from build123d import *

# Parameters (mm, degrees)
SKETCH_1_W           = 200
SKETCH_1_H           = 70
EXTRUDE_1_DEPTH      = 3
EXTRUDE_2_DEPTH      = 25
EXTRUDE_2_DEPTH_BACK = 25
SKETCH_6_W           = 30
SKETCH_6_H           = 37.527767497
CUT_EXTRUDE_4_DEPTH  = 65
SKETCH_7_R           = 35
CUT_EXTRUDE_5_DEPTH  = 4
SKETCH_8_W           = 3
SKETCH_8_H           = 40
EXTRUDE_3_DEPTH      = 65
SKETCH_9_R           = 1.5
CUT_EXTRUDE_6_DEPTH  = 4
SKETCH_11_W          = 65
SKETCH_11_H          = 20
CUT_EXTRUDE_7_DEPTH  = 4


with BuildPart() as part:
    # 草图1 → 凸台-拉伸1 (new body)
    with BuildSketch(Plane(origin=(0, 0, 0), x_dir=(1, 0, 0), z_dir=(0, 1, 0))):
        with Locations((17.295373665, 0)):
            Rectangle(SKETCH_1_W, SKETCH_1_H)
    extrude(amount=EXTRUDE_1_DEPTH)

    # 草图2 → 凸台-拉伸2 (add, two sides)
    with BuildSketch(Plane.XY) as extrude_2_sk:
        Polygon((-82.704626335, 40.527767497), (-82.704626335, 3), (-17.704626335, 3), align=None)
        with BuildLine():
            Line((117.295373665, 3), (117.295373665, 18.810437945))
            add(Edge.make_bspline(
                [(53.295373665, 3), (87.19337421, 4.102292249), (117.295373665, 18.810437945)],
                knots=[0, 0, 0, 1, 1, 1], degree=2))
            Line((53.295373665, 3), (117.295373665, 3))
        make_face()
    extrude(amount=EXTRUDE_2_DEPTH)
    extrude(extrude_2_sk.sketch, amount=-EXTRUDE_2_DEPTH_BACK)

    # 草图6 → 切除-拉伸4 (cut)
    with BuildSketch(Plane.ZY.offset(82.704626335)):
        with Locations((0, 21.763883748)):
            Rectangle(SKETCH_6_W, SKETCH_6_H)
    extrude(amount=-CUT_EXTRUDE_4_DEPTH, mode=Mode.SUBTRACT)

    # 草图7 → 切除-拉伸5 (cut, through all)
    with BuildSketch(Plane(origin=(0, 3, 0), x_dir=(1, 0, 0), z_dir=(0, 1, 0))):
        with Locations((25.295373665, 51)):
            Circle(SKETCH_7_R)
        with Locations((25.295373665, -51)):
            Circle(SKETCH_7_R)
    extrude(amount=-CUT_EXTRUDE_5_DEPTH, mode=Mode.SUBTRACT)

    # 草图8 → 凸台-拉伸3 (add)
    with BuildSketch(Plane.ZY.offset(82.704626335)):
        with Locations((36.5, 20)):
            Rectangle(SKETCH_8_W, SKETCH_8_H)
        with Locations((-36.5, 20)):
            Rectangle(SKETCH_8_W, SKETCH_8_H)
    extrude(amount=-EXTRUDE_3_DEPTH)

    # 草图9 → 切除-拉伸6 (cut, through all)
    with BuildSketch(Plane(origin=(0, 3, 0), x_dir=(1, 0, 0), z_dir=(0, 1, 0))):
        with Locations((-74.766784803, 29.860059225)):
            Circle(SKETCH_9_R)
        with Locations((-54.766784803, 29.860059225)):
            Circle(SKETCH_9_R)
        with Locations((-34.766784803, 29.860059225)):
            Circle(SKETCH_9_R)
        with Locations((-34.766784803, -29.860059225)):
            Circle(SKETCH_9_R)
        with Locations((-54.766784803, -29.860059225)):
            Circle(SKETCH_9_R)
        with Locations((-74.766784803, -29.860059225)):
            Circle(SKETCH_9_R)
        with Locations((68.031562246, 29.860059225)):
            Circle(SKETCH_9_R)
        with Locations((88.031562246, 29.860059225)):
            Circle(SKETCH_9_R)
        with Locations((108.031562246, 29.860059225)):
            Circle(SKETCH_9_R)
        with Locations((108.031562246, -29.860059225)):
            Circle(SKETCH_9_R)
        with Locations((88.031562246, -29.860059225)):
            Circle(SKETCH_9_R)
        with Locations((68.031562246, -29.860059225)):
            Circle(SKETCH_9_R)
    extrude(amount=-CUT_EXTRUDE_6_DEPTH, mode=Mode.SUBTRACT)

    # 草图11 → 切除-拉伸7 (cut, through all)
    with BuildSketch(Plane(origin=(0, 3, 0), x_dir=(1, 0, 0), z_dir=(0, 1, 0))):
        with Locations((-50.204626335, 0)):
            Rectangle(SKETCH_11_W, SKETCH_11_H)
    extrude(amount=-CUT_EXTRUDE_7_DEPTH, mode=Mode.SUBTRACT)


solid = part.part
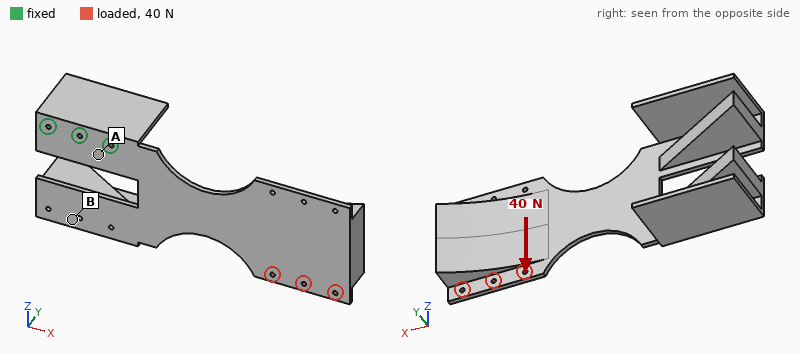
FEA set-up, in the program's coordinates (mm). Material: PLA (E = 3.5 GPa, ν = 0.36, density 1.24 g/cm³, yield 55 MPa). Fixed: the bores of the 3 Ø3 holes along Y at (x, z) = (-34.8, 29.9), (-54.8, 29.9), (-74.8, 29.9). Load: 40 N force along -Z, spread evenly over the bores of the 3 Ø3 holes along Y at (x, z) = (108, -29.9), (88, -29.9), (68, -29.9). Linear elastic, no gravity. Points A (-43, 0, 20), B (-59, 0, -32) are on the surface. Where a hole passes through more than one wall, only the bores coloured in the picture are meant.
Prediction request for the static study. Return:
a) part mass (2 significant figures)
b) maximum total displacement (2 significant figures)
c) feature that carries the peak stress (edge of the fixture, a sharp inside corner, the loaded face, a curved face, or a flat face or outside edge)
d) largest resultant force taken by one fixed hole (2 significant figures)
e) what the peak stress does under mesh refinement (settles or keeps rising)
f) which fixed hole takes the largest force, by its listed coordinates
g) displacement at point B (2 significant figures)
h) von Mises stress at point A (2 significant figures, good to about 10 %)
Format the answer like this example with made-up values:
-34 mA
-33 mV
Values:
110 g
2.3 mm
edge of the fixture
200 N
keeps rising
(-34.8, 29.9)
0.85 mm
3.9 MPa
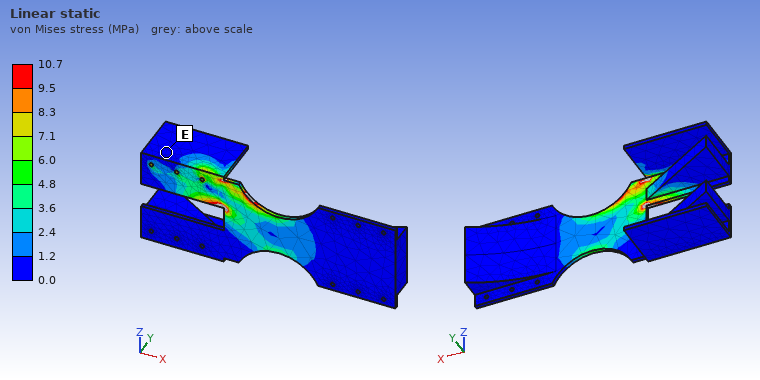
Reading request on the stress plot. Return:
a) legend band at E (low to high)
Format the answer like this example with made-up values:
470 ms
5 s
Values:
0.0 to 1.2 MPa
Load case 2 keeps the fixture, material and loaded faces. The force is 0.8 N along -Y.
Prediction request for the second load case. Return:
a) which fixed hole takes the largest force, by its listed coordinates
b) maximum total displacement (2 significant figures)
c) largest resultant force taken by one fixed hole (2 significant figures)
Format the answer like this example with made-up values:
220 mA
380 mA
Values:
(-34.8, 29.9)
2.4 mm
3.8 N
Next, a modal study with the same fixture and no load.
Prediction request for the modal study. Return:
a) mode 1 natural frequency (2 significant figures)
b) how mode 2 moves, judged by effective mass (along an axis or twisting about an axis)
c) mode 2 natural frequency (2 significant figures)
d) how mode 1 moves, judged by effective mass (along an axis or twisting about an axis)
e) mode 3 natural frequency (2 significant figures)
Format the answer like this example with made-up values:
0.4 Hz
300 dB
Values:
17 Hz
along Y
38 Hz
along Y
75 Hz
